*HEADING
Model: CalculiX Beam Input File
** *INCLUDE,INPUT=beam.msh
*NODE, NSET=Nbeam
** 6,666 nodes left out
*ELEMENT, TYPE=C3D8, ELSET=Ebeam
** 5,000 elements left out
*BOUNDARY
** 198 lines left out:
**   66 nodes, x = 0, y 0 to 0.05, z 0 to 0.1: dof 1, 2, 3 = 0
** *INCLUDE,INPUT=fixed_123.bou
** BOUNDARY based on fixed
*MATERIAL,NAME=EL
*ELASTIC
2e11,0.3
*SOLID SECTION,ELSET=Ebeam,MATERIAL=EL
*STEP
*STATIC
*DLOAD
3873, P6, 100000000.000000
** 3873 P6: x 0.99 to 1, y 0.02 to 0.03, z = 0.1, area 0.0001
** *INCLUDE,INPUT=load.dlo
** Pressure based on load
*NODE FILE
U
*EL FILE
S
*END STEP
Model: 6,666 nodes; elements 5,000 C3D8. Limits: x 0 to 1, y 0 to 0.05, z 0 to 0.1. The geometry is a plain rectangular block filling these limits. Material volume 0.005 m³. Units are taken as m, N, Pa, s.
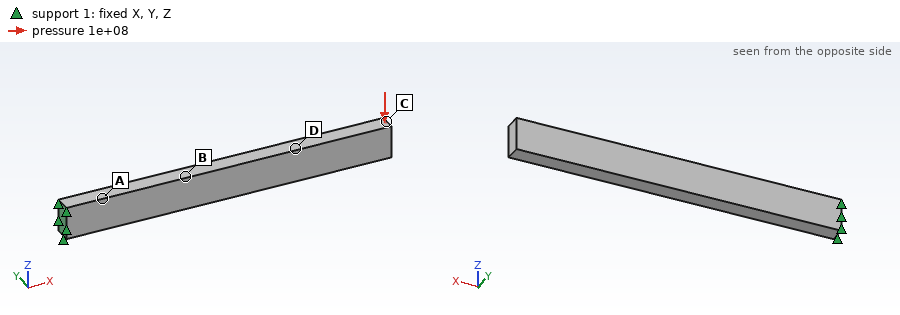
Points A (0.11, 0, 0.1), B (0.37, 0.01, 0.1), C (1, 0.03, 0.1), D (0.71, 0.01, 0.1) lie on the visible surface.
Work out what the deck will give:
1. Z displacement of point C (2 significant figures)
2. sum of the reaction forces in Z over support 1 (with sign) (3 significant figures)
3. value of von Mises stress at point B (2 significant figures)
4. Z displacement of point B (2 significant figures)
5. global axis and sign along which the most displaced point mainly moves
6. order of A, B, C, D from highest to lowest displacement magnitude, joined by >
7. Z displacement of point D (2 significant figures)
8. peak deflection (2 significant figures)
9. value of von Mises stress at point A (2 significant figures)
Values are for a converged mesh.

-0.0040 m
10000 N
7.5e+07 Pa
-7.2e-04 m
-Z
C > D > B > A
-0.0023 m
0.0040 m
1.1e+08 Pa
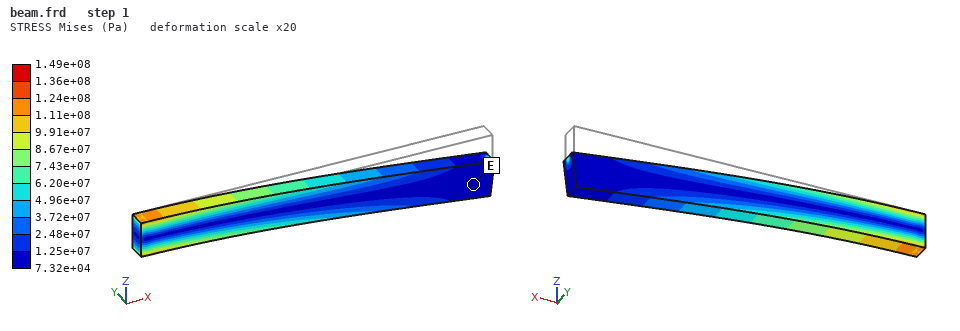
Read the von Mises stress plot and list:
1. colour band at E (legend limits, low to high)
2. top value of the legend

7.32e+04 to 1.25e+07 Pa
1.49e+08 Pa
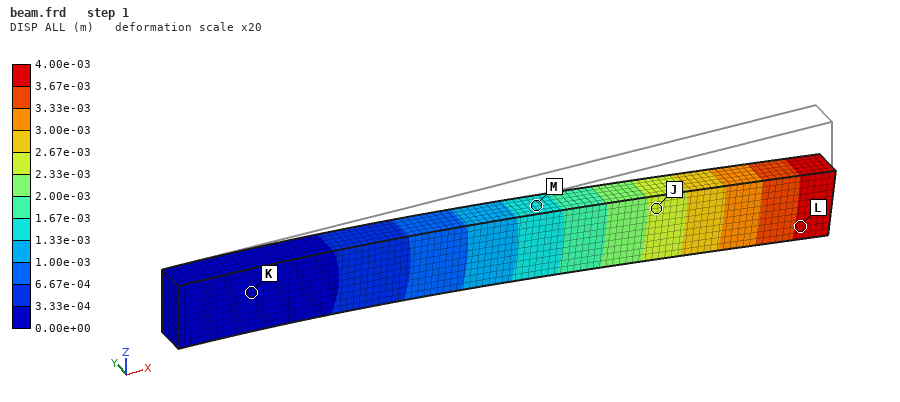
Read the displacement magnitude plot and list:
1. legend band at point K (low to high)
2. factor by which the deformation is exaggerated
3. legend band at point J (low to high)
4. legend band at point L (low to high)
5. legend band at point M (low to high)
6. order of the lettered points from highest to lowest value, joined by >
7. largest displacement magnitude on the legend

0.00e+00 to 3.33e-04 m
20
2.33e-03 to 2.67e-03 m
3.67e-03 to 4.00e-03 m
1.33e-03 to 1.67e-03 m
L > J > M > K
4.00e-03 m
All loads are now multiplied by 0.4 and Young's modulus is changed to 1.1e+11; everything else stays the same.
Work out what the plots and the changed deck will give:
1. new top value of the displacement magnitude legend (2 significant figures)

0.0029 m
